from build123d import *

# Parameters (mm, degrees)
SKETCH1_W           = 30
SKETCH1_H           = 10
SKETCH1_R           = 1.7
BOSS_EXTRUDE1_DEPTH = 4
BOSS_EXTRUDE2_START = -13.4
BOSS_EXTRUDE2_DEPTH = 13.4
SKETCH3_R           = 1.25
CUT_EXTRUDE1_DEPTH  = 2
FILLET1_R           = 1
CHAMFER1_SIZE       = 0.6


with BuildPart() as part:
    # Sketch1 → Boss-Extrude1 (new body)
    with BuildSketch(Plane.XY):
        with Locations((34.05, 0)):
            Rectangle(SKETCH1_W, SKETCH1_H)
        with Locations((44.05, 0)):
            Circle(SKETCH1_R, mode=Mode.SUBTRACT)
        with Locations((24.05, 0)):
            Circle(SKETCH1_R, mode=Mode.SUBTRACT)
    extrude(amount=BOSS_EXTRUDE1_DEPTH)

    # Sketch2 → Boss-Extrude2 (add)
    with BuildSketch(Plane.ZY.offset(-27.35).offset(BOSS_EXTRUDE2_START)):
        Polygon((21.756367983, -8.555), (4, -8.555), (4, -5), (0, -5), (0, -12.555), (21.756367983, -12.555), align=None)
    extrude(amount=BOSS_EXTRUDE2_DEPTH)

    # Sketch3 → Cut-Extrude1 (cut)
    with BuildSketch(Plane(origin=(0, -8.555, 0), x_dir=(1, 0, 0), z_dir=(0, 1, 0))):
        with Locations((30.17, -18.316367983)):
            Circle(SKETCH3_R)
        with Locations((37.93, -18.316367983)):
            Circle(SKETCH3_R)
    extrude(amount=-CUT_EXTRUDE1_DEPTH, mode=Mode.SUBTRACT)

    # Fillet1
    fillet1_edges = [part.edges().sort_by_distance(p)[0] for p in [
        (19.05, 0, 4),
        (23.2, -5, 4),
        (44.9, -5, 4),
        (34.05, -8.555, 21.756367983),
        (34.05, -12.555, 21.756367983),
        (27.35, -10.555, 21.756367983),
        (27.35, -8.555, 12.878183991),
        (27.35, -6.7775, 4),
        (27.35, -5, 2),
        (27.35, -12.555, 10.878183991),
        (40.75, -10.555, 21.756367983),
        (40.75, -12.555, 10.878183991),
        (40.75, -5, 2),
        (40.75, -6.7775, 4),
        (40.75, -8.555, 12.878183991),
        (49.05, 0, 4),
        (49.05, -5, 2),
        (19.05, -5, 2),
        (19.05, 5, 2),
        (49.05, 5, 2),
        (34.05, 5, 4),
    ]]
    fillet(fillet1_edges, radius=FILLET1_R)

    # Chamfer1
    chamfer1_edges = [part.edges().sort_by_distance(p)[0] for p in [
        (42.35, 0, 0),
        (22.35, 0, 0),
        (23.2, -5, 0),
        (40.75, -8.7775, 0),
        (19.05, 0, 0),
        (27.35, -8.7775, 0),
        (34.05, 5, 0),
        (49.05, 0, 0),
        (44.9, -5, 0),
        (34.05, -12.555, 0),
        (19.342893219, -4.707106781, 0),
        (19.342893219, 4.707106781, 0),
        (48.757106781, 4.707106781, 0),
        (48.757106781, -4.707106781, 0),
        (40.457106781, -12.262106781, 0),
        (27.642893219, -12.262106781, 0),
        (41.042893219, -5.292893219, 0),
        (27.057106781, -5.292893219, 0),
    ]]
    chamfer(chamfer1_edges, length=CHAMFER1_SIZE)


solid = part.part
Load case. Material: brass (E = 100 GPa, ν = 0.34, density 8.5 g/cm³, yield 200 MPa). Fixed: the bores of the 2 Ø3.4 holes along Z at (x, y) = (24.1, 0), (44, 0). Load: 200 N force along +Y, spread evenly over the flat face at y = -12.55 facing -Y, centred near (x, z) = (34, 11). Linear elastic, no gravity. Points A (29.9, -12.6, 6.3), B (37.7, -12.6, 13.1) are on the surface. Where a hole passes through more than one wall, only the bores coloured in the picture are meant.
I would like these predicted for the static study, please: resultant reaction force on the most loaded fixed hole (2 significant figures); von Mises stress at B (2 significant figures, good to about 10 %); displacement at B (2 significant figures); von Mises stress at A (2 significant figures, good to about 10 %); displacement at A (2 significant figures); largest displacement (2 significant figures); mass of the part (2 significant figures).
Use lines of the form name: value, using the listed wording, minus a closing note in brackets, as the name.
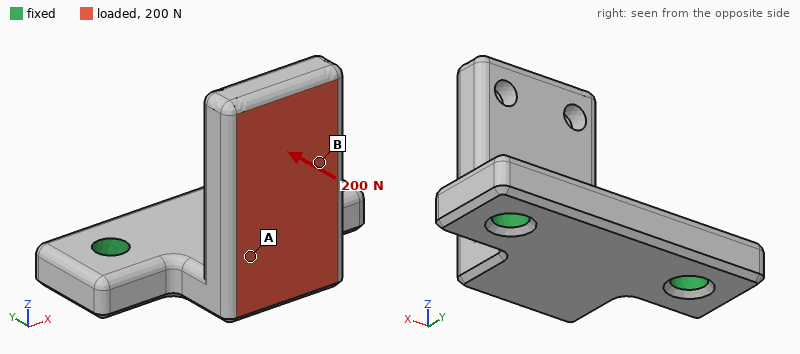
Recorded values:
resultant reaction force on the most loaded fixed hole: 110 N
von Mises stress at B: 9.1 MPa
displacement at B: 44 µm
von Mises stress at A: 30 MPa
displacement at A: 25 µm
largest displacement: 73 µm
mass of the part: 20 g
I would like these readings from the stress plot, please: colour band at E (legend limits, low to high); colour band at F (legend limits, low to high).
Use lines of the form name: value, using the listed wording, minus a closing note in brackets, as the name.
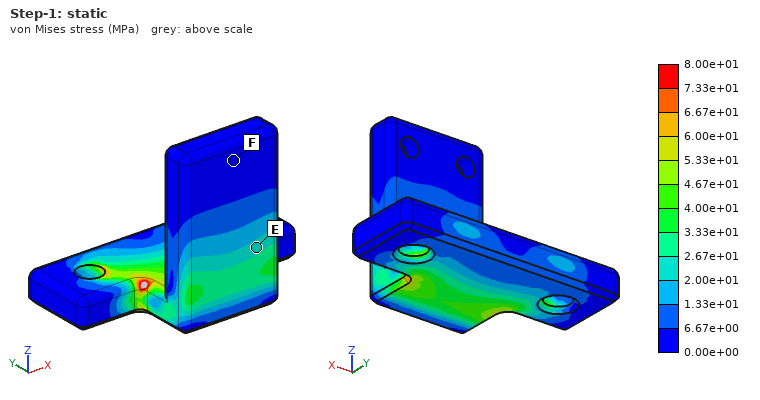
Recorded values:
colour band at E: 2.00e+01 to 2.67e+01 MPa
colour band at F: 0.00e+00 to 6.67e+00 MPa
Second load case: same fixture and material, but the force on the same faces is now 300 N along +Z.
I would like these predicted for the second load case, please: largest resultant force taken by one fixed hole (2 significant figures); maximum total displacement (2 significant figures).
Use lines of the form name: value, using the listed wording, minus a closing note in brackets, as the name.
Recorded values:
largest resultant force taken by one fixed hole: 150 N
maximum total displacement: 87 µm
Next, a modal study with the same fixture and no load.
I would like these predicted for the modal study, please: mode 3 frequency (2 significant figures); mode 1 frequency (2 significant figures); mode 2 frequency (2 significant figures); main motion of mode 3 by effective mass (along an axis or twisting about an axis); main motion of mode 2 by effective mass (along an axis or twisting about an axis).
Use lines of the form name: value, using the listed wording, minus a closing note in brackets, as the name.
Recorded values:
mode 3 frequency: 8800 Hz
mode 1 frequency: 3100 Hz
mode 2 frequency: 5500 Hz
main motion of mode 3 by effective mass: along Z
main motion of mode 2 by effective mass: along X
